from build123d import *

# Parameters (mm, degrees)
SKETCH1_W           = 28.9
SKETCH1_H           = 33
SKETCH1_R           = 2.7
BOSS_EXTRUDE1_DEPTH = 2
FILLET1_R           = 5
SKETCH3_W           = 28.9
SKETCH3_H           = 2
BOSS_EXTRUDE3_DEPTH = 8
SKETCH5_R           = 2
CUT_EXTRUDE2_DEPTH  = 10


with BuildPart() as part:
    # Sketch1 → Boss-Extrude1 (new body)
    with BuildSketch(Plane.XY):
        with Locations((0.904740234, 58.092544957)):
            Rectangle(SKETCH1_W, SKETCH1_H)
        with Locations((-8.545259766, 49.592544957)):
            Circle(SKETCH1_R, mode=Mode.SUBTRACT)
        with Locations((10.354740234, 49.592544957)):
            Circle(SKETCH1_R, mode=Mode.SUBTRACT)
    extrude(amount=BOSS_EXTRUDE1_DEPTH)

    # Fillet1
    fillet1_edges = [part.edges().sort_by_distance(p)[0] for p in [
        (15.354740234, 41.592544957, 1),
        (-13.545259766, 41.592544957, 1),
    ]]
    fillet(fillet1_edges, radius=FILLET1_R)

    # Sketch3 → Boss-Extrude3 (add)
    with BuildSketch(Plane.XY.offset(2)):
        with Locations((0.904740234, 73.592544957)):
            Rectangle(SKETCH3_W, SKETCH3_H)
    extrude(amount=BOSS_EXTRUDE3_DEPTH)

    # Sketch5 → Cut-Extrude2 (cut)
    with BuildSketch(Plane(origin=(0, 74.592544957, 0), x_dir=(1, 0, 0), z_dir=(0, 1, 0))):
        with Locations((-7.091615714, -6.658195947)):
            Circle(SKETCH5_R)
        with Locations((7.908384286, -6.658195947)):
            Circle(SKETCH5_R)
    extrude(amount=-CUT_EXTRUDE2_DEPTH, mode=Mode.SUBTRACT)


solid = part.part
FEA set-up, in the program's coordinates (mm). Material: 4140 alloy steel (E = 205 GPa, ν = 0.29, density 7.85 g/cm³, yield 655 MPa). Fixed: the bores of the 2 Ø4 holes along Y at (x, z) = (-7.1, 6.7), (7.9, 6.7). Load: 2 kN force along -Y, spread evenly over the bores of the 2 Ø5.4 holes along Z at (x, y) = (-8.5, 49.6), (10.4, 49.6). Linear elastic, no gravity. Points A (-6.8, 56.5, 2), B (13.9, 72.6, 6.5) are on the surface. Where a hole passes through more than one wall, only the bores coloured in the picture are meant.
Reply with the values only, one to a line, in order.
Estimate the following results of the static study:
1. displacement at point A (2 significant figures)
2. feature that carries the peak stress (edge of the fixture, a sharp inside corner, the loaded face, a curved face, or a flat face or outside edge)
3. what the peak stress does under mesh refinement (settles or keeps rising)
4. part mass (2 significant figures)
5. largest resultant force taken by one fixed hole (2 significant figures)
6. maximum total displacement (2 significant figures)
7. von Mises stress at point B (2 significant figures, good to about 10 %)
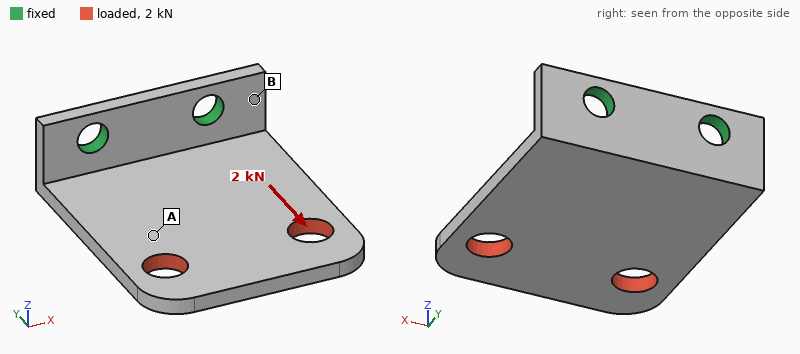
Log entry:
0.10 mm
edge of the fixture
keeps rising
17 g
1.1 kN
0.19 mm
130 MPa
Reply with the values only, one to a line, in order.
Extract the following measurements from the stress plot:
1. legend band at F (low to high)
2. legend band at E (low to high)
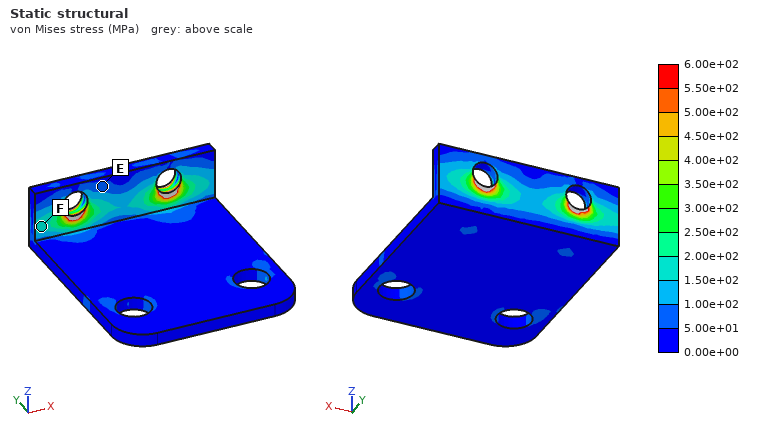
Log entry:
1.50e+02 to 2.00e+02 MPa
5.00e+01 to 1.00e+02 MPa
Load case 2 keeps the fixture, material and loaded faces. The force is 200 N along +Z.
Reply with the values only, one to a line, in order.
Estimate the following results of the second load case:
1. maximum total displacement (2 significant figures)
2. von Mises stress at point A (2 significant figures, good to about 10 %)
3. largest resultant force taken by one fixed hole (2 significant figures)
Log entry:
0.49 mm
69 MPa
110 N
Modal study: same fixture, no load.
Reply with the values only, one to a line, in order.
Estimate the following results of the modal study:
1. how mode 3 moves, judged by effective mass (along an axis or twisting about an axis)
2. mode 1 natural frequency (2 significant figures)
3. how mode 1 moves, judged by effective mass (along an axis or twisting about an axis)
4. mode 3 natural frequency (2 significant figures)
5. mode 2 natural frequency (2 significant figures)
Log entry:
along X
1400 Hz
along Z
6500 Hz
4100 Hz
